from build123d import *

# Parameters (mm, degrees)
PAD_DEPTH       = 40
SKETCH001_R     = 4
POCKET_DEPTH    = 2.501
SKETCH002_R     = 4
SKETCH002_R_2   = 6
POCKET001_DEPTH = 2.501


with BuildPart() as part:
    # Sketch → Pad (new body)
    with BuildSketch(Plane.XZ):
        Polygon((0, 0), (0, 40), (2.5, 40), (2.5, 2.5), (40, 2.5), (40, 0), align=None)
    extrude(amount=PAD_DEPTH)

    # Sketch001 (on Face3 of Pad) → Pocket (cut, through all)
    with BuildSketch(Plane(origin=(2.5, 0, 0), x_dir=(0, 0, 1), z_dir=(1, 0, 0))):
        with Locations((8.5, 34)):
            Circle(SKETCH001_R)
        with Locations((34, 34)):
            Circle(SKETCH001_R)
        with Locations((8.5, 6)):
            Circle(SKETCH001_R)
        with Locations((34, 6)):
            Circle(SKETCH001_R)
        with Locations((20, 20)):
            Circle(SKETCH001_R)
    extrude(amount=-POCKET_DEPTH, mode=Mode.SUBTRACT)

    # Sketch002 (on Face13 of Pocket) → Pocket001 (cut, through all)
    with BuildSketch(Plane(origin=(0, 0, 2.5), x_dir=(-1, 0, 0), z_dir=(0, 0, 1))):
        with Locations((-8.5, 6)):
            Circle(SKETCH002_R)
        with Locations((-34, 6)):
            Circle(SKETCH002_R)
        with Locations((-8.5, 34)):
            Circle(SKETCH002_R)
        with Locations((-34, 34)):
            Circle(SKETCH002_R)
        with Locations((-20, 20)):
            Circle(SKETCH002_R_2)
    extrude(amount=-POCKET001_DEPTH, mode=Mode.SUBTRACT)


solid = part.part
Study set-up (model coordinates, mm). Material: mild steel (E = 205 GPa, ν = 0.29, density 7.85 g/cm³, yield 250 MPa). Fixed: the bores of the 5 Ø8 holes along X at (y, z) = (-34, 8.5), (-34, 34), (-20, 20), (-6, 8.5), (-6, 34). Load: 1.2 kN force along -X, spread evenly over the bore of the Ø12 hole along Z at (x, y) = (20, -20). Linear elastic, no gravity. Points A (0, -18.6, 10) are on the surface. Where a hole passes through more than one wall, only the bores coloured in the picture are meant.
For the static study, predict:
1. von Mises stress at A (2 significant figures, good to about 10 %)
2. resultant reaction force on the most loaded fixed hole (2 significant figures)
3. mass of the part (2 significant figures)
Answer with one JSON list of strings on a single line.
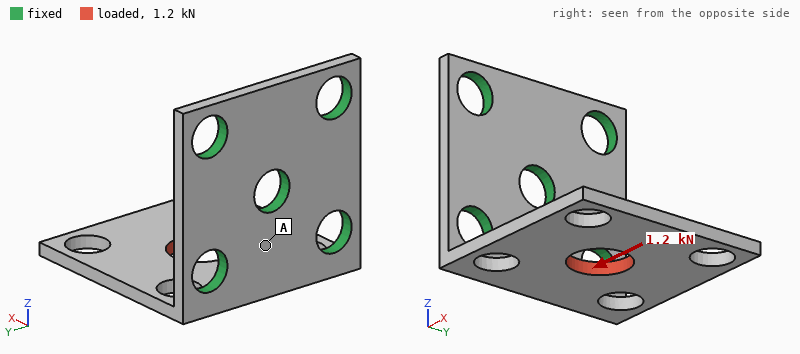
["17 MPa", "630 N", "50 g"]
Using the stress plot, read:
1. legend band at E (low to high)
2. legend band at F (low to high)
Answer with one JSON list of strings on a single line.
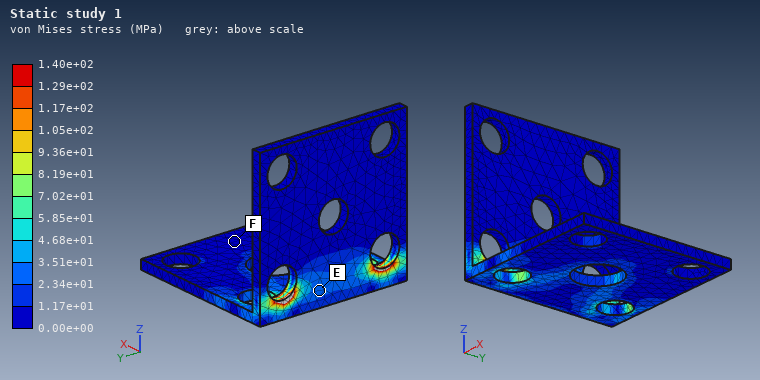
["2.34e+01 to 3.51e+01 MPa", "0.00e+00 to 1.17e+01 MPa"]
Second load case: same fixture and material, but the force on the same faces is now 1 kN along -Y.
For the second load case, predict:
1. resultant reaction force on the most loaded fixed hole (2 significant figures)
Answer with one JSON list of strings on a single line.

["820 N"]
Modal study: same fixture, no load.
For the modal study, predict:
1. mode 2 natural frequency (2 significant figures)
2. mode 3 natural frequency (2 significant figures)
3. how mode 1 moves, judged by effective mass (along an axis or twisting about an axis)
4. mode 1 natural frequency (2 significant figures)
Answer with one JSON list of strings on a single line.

["2900 Hz", "7000 Hz", "along Z", "1100 Hz"]
